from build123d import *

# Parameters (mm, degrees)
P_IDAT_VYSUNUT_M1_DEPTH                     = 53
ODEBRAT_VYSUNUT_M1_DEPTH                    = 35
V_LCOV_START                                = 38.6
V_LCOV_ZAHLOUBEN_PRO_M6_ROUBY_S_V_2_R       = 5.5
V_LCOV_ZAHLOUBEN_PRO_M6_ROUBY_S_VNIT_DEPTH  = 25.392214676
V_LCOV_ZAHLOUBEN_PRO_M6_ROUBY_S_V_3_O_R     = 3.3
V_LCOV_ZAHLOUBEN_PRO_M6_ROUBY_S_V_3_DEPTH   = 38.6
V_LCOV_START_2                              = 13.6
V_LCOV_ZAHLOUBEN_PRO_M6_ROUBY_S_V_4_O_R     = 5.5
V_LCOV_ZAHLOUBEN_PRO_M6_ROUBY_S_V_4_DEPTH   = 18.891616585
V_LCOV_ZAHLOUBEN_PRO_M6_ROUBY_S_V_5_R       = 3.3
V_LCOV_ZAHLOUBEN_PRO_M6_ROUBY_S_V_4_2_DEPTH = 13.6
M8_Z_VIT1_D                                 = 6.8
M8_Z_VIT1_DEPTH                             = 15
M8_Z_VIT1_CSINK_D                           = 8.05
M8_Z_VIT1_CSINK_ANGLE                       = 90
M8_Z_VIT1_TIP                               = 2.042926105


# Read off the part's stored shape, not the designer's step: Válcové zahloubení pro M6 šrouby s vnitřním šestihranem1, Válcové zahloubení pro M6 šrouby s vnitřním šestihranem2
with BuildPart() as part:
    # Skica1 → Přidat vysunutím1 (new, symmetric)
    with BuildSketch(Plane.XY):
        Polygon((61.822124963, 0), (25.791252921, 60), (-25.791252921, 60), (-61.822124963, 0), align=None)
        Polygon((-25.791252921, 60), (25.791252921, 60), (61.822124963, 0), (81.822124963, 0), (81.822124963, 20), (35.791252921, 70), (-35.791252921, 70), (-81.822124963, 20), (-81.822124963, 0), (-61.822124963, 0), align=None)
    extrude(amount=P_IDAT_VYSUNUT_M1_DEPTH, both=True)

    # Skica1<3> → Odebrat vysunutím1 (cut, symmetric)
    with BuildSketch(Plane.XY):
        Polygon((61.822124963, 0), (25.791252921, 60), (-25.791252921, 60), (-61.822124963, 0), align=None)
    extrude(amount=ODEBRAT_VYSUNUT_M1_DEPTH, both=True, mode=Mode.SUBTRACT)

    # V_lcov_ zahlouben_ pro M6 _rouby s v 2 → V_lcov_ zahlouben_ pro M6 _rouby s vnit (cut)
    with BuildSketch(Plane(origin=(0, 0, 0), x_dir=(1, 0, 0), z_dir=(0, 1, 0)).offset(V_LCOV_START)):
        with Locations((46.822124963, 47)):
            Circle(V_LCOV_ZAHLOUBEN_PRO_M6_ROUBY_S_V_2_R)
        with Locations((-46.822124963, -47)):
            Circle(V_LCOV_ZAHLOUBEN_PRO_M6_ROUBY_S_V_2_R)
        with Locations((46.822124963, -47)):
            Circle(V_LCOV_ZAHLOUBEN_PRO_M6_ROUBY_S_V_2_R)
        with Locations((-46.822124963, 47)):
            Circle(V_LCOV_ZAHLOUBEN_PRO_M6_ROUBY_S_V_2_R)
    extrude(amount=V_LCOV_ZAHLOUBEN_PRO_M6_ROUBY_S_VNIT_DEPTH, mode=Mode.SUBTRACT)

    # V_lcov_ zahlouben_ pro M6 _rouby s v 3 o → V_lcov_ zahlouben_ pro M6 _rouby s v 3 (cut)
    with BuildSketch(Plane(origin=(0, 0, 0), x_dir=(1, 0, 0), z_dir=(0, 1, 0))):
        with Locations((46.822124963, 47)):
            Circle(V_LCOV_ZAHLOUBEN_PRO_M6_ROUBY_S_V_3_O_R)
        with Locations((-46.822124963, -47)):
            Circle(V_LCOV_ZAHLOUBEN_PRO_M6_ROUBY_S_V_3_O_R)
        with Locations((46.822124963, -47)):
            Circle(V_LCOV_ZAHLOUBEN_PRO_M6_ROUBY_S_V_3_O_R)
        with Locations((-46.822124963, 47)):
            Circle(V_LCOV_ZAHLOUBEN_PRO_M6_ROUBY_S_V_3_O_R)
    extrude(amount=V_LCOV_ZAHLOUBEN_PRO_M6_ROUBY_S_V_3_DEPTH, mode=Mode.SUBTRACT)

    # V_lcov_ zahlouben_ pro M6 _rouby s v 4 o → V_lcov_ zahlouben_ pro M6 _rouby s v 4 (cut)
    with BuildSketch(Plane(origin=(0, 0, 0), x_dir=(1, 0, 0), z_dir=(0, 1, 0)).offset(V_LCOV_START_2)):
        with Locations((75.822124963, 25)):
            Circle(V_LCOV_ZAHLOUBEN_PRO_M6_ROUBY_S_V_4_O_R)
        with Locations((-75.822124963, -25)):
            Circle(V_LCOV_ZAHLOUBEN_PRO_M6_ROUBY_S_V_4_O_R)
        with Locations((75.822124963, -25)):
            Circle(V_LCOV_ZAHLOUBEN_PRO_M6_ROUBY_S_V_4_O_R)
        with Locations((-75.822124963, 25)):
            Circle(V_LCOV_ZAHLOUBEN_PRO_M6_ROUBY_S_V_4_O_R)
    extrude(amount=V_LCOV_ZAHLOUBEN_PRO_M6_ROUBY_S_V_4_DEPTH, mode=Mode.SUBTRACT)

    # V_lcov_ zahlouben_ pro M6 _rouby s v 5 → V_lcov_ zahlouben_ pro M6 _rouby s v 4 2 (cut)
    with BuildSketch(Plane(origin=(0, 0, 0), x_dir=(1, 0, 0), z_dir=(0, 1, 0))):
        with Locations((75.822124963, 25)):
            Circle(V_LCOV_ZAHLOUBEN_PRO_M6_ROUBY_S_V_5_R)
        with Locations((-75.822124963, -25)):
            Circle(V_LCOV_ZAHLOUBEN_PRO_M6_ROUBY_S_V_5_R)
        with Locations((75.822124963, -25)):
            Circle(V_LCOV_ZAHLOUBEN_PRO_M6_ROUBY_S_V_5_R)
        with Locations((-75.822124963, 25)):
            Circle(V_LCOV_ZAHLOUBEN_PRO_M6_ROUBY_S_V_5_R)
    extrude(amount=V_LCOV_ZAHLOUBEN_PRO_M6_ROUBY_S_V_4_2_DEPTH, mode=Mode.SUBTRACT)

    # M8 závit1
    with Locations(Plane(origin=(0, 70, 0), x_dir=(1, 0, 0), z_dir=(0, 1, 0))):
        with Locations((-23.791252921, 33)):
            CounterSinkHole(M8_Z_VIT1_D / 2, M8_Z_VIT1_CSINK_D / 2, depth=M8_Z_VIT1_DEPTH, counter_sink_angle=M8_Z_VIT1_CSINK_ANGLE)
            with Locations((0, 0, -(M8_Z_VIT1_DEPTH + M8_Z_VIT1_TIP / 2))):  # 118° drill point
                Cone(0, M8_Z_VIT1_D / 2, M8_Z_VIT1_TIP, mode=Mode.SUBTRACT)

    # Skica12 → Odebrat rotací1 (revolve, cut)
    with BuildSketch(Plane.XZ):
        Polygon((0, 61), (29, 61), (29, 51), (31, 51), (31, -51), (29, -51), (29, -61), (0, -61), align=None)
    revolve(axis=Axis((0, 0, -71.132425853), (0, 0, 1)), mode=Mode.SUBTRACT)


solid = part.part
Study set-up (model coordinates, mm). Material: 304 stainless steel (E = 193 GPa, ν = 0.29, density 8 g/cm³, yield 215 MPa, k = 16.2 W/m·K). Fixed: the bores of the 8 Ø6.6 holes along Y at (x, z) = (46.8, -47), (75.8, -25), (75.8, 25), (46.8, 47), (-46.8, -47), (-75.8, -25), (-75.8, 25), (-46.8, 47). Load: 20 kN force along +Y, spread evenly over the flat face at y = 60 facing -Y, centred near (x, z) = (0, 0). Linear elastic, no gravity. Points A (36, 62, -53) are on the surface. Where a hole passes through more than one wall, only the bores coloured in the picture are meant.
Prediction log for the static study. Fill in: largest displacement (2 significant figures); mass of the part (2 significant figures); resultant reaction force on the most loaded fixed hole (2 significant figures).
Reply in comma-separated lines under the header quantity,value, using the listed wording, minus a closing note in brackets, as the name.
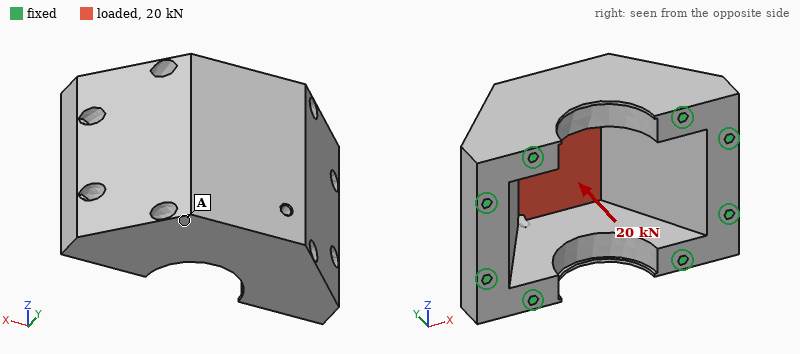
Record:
quantity,value
largest displacement,16 µm
mass of the part,4.2 kg
resultant reaction force on the most loaded fixed hole,4.8 kN
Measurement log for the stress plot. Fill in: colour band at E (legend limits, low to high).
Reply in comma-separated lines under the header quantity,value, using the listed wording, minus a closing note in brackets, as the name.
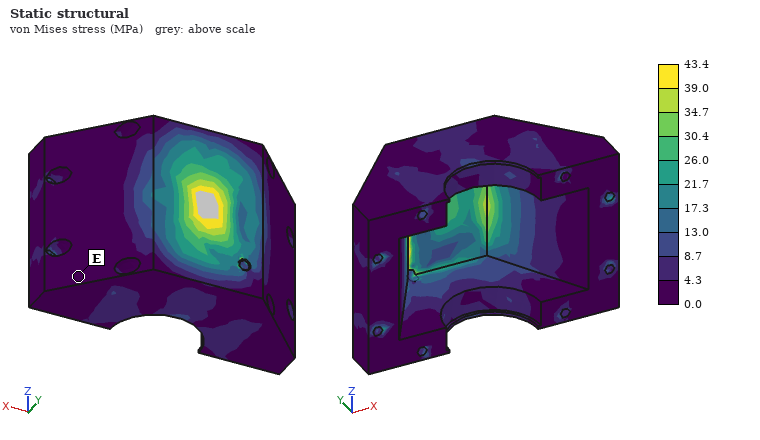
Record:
quantity,value
colour band at E,0.0 to 4.3 MPa
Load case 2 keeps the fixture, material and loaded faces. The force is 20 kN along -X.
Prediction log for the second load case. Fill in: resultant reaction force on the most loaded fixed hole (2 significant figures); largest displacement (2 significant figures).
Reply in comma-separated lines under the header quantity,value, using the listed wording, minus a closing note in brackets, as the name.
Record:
quantity,value
resultant reaction force on the most loaded fixed hole,4.8 kN
largest displacement,8.3 µm
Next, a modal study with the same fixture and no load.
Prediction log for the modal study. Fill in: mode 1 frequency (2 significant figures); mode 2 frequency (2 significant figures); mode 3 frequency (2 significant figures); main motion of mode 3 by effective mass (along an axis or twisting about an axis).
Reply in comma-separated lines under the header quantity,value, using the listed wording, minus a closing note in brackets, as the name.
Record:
quantity,value
mode 1 frequency,9200 Hz
mode 2 frequency,9200 Hz
mode 3 frequency,11 kHz
main motion of mode 3 by effective mass,along Y
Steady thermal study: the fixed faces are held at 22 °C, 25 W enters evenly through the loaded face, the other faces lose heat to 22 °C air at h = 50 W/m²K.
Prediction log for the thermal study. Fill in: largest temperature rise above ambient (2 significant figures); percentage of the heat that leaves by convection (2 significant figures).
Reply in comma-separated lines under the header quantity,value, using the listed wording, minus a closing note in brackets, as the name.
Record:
quantity,value
largest temperature rise above ambient,23 K
percentage of the heat that leaves by convection,54 %
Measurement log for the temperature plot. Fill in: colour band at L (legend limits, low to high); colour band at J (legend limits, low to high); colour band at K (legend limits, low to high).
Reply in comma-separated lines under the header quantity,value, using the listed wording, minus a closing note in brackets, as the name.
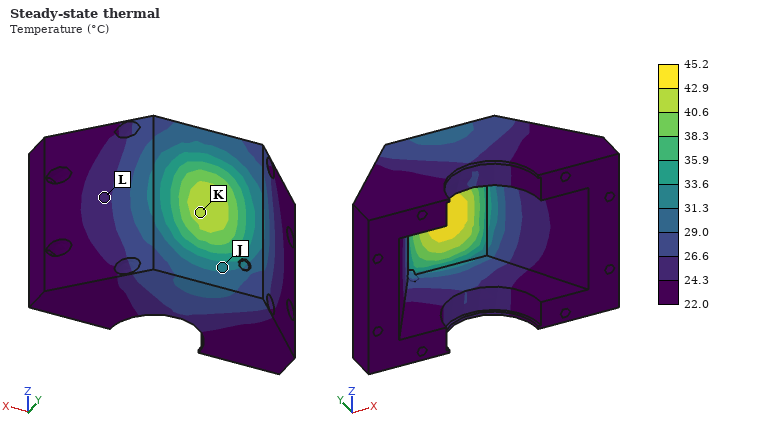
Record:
quantity,value
colour band at L,24.3 to 26.6 °C
colour band at J,31.3 to 33.6 °C
colour band at K,40.6 to 42.9 °C
